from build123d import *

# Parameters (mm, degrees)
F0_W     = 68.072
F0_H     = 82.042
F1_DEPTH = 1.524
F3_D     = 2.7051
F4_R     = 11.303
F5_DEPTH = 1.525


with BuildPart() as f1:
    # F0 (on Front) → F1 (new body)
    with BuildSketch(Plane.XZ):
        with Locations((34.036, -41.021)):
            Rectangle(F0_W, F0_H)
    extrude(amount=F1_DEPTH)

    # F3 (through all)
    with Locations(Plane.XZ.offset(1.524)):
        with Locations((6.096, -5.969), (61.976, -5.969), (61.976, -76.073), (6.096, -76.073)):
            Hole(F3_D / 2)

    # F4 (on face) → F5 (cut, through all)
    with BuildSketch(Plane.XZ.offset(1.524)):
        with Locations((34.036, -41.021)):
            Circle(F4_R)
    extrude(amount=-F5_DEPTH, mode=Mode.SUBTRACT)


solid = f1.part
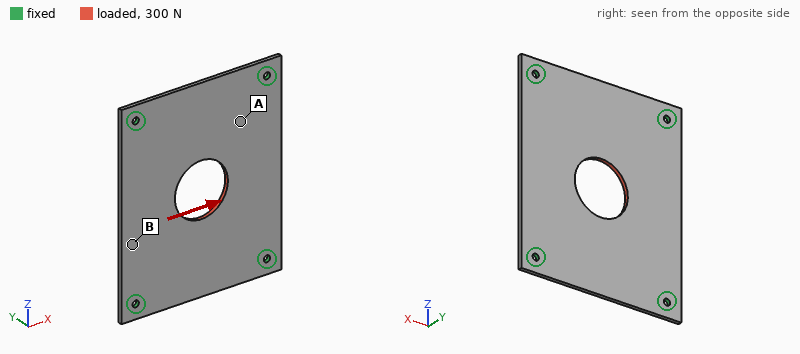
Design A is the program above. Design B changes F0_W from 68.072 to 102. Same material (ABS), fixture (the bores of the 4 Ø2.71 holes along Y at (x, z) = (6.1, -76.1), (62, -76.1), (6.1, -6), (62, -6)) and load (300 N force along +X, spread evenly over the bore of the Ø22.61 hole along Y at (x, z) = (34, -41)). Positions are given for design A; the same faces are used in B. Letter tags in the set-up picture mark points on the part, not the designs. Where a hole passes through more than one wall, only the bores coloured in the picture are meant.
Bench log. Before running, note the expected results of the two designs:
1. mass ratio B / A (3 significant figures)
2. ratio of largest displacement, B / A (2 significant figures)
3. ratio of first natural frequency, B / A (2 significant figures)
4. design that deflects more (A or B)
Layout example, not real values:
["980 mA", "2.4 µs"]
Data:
["1.54", "0.74", "0.96", "A"]
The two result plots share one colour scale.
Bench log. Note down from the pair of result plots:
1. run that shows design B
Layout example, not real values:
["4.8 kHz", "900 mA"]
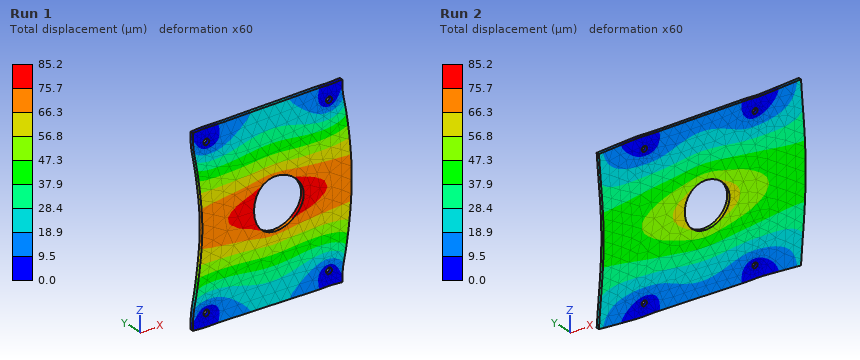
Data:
["Run 2"]
